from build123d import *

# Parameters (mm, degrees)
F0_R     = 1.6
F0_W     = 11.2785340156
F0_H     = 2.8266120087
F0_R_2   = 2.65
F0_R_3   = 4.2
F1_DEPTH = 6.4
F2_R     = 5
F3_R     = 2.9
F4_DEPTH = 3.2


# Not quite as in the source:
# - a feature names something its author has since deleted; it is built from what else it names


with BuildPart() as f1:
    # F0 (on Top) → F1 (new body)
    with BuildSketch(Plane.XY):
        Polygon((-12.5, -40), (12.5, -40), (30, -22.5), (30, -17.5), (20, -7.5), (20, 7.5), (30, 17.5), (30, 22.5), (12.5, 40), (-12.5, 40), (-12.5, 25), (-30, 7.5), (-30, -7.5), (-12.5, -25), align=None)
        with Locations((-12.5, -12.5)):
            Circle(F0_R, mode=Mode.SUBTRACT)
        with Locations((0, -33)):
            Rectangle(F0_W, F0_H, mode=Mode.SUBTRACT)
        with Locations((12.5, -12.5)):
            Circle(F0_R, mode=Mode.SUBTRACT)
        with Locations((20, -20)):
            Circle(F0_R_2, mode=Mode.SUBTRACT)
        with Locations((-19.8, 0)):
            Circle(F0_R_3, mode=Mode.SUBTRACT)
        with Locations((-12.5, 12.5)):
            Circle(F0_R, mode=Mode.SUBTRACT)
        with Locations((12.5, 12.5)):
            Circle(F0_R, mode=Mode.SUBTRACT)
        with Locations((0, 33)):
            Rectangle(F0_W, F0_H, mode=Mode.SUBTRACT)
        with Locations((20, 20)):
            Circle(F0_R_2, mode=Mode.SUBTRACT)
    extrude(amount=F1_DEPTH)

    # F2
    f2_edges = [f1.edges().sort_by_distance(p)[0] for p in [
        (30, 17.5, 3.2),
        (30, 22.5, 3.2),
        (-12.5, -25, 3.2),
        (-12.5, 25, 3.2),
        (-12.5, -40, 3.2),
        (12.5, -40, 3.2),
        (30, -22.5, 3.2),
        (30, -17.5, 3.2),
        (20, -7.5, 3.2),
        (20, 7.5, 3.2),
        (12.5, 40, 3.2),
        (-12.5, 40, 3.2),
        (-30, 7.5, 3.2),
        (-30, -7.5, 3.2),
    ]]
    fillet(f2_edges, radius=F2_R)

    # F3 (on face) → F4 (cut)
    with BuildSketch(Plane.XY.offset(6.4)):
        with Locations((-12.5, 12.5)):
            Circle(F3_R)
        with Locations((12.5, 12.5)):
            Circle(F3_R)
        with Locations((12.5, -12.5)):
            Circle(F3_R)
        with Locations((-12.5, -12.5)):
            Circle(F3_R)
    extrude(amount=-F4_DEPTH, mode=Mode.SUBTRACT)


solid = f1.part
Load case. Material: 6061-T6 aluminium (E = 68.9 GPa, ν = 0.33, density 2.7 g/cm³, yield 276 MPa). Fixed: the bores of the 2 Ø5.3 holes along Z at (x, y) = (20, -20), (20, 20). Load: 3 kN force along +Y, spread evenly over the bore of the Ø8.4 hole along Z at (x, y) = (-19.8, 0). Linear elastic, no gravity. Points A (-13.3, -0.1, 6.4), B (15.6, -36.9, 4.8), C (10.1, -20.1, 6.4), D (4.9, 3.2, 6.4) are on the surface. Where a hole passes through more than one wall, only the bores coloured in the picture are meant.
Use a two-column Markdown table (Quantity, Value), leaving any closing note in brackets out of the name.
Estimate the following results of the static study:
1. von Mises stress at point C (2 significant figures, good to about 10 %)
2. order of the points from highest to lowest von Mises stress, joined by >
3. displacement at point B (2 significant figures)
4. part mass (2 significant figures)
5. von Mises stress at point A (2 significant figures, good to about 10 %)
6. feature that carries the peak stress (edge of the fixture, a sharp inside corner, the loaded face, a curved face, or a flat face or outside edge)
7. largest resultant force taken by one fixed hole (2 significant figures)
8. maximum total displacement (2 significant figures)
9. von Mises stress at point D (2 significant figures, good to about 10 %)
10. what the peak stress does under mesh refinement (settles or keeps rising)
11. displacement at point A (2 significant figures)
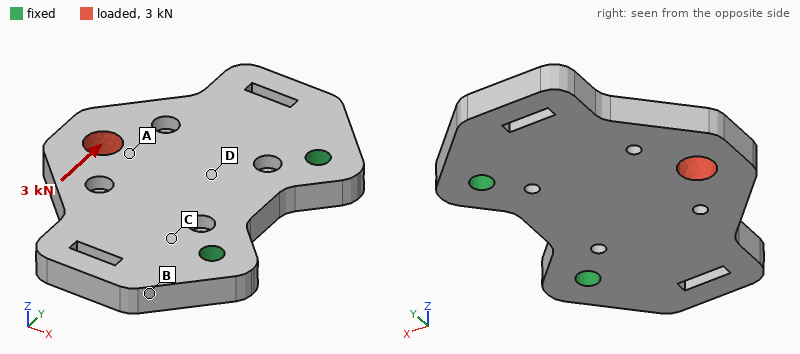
| Quantity | Value |
|---|---|
| von Mises stress at point C | 23 MPa |
| order of the points from highest to lowest von Mises stress, joined by > | A > C > D > B |
| displacement at point B | 14 µm |
| part mass | 55 g |
| von Mises stress at point A | 37 MPa |
| feature that carries the peak stress | edge of the fixture |
| largest resultant force taken by one fixed hole | 3.1 kN |
| maximum total displacement | 34 µm |
| von Mises stress at point D | 18 MPa |
| what the peak stress does under mesh refinement | keeps rising |
| displacement at point A | 23 µm |
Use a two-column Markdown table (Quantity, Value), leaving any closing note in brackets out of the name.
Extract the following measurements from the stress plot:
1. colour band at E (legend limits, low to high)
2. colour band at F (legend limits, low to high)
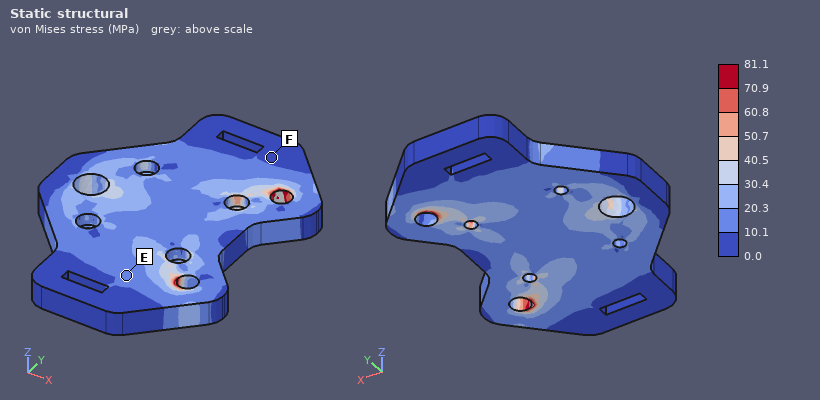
| Quantity | Value |
|---|---|
| colour band at E | 10.1 to 20.3 MPa |
| colour band at F | 0.0 to 10.1 MPa |
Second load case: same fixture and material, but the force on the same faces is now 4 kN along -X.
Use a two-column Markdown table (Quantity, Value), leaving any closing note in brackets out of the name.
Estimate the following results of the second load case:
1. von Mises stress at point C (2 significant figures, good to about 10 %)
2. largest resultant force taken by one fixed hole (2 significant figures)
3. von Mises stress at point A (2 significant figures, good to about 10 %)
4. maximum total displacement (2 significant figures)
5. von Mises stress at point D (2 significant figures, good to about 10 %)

| Quantity | Value |
|---|---|
| von Mises stress at point C | 18 MPa |
| largest resultant force taken by one fixed hole | 2.1 kN |
| von Mises stress at point A | 24 MPa |
| maximum total displacement | 19 µm |
| von Mises stress at point D | 12 MPa |
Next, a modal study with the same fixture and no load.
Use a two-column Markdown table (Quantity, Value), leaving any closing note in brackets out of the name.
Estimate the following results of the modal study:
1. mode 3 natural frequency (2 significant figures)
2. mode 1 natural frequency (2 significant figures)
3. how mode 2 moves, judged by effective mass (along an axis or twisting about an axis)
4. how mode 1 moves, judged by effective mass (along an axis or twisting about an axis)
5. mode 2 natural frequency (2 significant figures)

| Quantity | Value |
|---|---|
| mode 3 natural frequency | 7700 Hz |
| mode 1 natural frequency | 2500 Hz |
| how mode 2 moves, judged by effective mass | twisting about X |
| how mode 1 moves, judged by effective mass | along Z |
| mode 2 natural frequency | 5200 Hz |
